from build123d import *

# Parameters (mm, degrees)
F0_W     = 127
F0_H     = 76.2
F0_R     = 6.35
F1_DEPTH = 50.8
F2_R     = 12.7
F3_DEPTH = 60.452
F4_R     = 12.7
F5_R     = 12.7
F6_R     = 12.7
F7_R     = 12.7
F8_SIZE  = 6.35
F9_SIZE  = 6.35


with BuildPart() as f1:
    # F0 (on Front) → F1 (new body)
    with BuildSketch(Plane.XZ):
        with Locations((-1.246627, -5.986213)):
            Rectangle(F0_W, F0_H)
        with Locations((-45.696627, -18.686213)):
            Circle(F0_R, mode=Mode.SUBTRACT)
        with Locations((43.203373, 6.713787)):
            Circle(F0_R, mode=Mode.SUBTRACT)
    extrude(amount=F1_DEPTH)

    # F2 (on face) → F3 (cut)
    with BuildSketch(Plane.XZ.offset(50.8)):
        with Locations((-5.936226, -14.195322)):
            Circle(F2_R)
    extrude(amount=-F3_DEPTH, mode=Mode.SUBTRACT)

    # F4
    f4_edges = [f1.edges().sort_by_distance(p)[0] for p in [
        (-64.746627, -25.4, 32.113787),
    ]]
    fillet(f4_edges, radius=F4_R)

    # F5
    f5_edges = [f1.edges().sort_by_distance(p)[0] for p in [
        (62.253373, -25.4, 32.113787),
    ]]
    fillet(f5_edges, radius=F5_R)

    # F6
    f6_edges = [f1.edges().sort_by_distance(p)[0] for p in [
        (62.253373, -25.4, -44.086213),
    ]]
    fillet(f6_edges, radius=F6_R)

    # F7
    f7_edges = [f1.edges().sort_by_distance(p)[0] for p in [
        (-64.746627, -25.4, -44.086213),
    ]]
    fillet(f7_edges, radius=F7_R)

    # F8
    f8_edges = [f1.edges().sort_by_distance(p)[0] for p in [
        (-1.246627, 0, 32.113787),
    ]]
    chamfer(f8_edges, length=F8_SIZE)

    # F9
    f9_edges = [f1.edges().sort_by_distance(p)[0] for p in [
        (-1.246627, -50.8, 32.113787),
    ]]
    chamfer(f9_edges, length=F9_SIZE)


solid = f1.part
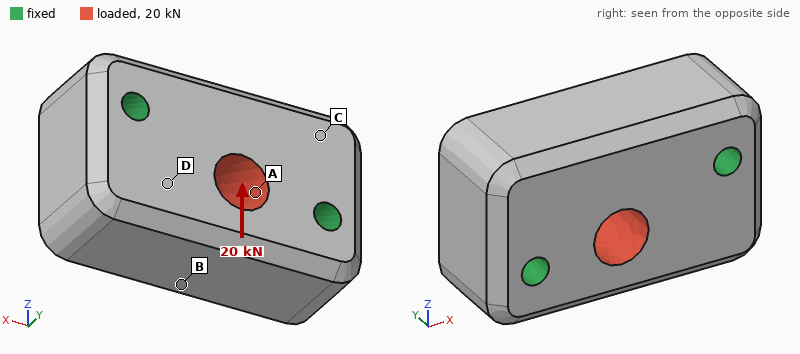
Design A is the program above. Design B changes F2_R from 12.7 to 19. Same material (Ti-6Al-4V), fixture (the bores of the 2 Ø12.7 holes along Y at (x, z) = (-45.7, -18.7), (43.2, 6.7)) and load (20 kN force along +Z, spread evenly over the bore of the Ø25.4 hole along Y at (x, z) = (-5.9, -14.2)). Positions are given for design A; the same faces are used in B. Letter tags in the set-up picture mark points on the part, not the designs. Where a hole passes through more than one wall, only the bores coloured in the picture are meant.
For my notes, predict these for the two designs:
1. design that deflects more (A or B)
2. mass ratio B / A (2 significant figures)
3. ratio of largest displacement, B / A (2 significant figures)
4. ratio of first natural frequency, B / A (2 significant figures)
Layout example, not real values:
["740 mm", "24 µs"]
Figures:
["B", "0.93", "1.1", "1.0"]
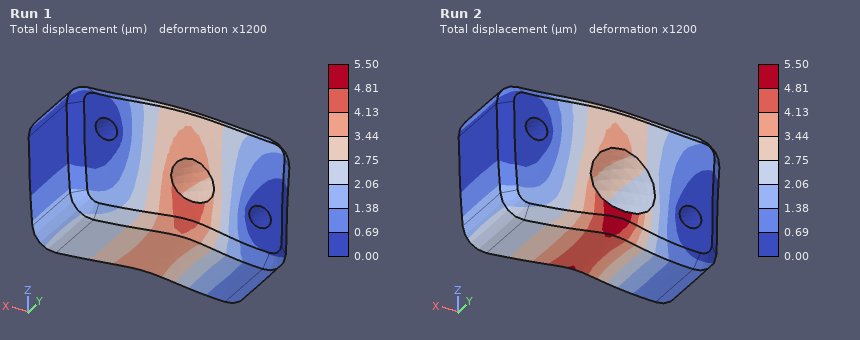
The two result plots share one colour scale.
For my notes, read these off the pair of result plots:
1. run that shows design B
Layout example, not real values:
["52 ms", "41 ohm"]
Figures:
["Run 2"]
